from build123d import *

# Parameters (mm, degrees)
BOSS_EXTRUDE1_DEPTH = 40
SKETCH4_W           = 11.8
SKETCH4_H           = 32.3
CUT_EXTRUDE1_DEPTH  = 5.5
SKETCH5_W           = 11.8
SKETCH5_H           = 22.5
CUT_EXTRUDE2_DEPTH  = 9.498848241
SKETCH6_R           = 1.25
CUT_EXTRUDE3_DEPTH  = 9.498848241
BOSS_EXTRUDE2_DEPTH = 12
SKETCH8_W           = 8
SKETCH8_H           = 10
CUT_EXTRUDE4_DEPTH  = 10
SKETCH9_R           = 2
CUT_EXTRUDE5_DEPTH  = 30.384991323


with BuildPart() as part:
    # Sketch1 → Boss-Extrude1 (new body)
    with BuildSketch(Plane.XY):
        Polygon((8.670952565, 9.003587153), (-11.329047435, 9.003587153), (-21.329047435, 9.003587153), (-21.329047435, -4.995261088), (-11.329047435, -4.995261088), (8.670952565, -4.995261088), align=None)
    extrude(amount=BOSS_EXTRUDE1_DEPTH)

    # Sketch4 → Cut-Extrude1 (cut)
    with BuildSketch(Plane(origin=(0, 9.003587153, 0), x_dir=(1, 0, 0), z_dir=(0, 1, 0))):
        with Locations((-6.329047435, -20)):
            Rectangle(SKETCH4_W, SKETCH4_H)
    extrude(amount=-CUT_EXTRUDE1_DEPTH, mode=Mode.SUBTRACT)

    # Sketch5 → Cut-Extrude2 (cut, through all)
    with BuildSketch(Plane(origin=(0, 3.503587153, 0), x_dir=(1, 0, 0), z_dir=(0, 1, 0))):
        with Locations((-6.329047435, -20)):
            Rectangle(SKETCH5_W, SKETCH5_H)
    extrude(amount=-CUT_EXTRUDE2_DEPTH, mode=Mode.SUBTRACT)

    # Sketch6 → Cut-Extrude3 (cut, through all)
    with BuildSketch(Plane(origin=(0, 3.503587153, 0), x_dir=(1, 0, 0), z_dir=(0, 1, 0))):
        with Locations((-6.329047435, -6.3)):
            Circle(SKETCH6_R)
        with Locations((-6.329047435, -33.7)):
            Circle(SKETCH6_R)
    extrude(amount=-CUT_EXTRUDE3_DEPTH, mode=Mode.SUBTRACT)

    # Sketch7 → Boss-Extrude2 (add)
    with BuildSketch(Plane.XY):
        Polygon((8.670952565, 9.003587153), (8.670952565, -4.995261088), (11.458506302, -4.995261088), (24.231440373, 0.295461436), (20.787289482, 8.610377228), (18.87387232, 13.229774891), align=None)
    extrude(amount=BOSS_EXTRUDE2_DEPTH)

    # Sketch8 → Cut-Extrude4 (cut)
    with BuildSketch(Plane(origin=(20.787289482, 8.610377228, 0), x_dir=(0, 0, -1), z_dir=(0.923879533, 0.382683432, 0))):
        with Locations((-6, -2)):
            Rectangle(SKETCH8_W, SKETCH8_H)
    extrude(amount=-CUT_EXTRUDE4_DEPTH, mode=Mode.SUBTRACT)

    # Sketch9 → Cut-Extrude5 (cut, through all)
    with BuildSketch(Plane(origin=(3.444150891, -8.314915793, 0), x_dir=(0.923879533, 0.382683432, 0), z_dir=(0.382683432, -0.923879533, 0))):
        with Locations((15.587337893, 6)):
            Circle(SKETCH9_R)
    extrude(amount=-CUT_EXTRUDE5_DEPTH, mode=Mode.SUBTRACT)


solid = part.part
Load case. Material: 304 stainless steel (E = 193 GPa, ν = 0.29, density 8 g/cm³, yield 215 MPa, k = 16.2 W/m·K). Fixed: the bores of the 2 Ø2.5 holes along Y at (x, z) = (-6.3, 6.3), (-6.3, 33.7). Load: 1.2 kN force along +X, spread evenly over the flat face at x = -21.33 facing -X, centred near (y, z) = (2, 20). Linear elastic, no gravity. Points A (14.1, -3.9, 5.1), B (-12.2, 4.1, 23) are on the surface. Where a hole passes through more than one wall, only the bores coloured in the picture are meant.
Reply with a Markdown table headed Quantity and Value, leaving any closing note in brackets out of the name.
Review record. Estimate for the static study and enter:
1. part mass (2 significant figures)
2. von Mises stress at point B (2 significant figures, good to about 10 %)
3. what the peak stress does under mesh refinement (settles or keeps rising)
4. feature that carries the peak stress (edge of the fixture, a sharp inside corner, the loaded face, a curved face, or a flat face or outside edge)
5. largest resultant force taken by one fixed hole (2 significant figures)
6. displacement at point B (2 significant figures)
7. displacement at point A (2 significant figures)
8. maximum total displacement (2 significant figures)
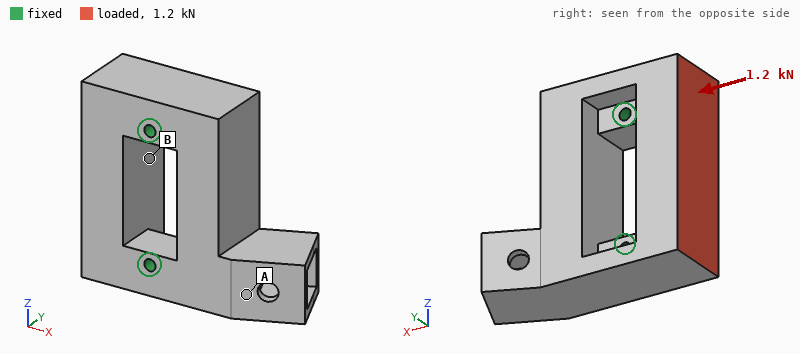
| Quantity | Value |
|---|---|
| part mass | 110 g |
| von Mises stress at point B | 6.7 MPa |
| what the peak stress does under mesh refinement | keeps rising |
| feature that carries the peak stress | edge of the fixture |
| largest resultant force taken by one fixed hole | 630 N |
| displacement at point B | 1.8 µm |
| displacement at point A | 1.0 µm |
| maximum total displacement | 2.8 µm |
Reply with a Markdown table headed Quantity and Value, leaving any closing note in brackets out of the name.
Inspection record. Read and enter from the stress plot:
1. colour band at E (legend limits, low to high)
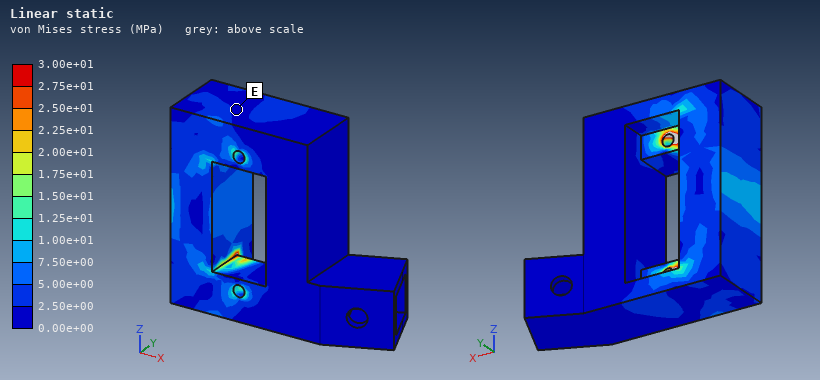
| Quantity | Value |
|---|---|
| colour band at E | 0.00e+00 to 2.50e+00 MPa |
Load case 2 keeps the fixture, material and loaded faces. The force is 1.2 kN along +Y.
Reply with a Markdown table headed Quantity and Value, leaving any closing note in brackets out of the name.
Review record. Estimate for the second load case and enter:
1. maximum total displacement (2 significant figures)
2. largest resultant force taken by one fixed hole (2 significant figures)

| Quantity | Value |
|---|---|
| maximum total displacement | 9.9 µm |
| largest resultant force taken by one fixed hole | 600 N |
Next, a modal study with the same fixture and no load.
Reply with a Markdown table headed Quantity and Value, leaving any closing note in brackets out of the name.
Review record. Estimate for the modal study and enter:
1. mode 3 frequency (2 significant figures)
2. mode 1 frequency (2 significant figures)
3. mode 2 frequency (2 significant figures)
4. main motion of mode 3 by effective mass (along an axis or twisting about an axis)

| Quantity | Value |
|---|---|
| mode 3 frequency | 14 kHz |
| mode 1 frequency | 8000 Hz |
| mode 2 frequency | 12 kHz |
| main motion of mode 3 by effective mass | along Y |
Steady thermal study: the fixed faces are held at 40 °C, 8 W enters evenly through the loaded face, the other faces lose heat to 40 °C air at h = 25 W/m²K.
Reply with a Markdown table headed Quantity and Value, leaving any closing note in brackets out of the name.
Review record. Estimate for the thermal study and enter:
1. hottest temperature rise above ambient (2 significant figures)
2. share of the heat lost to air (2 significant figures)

| Quantity | Value |
|---|---|
| hottest temperature rise above ambient | 34 K |
| share of the heat lost to air | 15 % |
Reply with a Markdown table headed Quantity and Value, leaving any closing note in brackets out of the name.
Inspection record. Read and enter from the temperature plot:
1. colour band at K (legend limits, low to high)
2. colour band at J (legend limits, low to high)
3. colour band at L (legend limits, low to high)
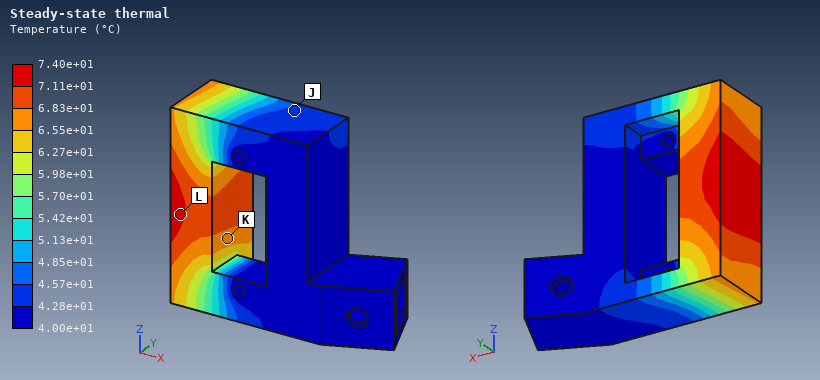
| Quantity | Value |
|---|---|
| colour band at K | 6.55e+01 to 6.83e+01 °C |
| colour band at J | 4.28e+01 to 4.57e+01 °C |
| colour band at L | 7.11e+01 to 7.40e+01 °C |
